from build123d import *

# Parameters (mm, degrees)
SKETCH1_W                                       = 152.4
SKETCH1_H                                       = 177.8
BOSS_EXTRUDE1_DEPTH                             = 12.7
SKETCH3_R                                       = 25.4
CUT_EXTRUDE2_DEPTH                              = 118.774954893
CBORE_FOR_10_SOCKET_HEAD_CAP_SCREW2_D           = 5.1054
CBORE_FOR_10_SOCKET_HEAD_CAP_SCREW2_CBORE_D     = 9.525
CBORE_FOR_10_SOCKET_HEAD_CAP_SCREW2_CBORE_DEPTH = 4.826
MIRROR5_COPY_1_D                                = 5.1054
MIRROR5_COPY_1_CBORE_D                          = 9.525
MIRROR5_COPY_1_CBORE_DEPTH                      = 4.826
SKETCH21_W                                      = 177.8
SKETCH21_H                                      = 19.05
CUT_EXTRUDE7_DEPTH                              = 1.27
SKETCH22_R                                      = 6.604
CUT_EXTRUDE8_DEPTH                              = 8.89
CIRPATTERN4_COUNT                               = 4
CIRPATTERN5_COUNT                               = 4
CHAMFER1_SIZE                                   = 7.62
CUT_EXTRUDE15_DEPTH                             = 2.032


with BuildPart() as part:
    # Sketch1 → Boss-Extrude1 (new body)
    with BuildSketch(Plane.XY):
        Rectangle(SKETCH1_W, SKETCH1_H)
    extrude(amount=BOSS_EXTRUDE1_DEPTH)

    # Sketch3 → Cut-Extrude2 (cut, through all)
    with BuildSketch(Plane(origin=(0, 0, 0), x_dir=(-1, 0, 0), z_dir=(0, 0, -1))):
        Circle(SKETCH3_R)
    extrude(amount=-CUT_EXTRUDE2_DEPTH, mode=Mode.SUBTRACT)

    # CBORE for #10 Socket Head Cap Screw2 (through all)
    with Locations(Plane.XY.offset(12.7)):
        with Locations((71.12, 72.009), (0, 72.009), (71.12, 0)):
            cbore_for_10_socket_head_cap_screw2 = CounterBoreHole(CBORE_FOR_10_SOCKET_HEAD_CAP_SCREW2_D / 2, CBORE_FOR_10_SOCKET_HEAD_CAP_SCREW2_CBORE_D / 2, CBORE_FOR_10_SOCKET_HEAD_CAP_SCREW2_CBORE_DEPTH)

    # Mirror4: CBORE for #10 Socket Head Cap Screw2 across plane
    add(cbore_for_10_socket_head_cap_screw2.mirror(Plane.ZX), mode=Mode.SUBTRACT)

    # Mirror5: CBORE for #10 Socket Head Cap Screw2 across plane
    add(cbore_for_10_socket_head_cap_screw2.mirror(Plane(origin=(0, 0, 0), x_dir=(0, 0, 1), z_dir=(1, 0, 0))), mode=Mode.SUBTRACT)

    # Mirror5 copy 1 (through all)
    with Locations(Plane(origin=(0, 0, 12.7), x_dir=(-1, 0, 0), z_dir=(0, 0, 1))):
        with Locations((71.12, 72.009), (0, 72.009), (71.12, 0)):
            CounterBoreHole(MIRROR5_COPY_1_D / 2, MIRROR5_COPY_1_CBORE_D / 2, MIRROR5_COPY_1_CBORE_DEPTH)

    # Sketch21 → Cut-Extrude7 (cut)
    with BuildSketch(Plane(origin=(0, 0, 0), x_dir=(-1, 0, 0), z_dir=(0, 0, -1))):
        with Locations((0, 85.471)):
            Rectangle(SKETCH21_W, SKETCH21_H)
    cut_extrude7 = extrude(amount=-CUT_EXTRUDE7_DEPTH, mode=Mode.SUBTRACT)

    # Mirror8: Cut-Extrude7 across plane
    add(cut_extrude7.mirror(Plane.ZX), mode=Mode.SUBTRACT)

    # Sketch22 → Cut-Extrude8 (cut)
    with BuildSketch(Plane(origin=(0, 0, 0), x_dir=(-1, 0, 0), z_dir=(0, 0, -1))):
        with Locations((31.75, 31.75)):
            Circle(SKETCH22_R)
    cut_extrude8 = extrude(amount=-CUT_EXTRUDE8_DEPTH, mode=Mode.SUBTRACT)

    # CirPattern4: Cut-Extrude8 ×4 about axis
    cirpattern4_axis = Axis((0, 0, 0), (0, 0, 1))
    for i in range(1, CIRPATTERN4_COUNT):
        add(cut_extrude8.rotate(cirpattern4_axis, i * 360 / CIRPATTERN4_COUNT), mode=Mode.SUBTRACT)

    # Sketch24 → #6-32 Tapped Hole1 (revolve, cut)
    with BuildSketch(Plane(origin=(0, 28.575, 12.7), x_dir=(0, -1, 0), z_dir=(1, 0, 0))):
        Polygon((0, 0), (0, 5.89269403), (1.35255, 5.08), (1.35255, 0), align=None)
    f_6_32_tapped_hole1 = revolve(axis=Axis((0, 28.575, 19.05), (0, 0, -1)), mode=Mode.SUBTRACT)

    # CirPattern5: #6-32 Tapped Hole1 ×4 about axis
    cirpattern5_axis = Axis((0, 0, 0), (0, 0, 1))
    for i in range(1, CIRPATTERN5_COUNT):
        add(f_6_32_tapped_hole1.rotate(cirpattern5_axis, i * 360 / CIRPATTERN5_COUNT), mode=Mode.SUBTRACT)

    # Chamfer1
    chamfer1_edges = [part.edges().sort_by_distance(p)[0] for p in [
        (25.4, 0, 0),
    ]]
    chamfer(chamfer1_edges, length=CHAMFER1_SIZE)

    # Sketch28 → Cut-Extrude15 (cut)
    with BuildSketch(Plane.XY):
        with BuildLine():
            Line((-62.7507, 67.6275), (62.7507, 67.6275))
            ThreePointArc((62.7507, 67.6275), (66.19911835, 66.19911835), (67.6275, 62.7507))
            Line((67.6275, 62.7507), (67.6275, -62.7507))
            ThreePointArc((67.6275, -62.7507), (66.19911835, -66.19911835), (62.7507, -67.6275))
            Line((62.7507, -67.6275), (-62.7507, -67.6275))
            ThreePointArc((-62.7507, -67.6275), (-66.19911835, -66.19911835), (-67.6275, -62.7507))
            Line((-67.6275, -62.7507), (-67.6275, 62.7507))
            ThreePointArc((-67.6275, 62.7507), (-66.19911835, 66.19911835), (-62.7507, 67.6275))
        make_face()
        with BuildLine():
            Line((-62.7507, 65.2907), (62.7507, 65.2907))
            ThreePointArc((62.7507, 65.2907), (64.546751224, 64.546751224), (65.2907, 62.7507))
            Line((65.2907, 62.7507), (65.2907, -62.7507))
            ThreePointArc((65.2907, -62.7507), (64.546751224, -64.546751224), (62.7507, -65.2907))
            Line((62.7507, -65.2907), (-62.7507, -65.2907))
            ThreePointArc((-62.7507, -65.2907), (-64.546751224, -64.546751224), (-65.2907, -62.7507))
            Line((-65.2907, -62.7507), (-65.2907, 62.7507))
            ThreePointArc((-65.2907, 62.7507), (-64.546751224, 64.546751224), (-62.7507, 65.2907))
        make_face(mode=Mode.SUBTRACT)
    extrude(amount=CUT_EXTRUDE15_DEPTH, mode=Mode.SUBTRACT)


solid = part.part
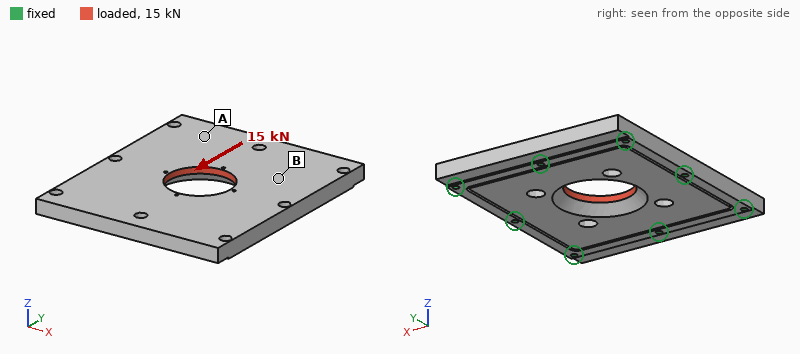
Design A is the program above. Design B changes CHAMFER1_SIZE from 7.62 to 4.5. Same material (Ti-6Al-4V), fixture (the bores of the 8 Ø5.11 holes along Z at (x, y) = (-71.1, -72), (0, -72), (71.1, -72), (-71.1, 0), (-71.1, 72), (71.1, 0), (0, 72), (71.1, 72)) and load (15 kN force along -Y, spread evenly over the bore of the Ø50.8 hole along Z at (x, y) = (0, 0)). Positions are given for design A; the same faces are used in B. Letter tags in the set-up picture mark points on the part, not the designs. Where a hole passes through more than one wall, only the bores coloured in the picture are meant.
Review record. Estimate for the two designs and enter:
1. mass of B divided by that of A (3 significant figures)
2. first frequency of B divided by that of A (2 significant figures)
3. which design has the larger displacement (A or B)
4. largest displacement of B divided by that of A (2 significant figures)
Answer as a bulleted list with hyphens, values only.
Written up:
- 1.01
- 0.98
- A
- 0.76
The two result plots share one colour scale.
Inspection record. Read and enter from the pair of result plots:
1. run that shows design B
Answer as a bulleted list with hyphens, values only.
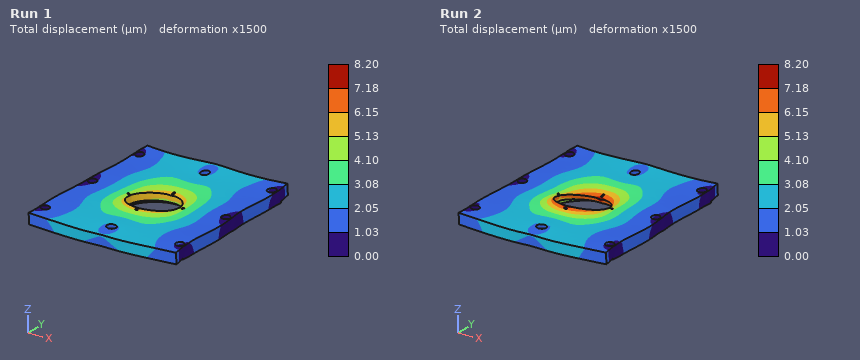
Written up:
- Run 1
